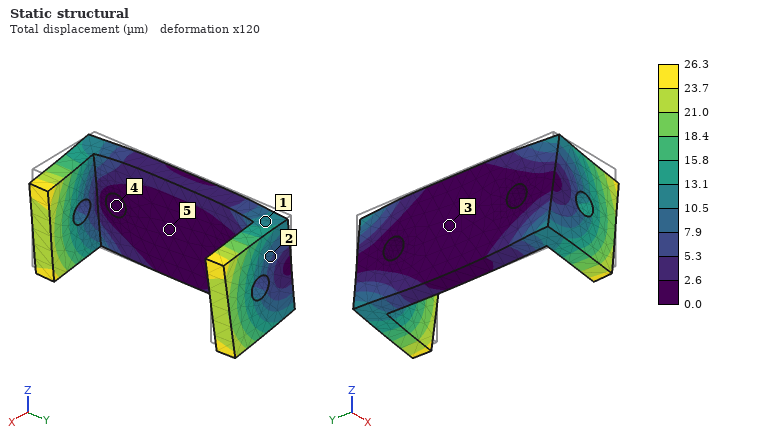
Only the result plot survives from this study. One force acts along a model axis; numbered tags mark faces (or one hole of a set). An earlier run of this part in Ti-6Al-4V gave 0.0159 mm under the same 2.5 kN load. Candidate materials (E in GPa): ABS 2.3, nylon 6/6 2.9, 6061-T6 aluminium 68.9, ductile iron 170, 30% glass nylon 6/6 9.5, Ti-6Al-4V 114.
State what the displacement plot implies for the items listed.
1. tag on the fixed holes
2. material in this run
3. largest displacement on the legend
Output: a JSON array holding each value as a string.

["4", "6061-T6 aluminium", "26.3 µm"]
